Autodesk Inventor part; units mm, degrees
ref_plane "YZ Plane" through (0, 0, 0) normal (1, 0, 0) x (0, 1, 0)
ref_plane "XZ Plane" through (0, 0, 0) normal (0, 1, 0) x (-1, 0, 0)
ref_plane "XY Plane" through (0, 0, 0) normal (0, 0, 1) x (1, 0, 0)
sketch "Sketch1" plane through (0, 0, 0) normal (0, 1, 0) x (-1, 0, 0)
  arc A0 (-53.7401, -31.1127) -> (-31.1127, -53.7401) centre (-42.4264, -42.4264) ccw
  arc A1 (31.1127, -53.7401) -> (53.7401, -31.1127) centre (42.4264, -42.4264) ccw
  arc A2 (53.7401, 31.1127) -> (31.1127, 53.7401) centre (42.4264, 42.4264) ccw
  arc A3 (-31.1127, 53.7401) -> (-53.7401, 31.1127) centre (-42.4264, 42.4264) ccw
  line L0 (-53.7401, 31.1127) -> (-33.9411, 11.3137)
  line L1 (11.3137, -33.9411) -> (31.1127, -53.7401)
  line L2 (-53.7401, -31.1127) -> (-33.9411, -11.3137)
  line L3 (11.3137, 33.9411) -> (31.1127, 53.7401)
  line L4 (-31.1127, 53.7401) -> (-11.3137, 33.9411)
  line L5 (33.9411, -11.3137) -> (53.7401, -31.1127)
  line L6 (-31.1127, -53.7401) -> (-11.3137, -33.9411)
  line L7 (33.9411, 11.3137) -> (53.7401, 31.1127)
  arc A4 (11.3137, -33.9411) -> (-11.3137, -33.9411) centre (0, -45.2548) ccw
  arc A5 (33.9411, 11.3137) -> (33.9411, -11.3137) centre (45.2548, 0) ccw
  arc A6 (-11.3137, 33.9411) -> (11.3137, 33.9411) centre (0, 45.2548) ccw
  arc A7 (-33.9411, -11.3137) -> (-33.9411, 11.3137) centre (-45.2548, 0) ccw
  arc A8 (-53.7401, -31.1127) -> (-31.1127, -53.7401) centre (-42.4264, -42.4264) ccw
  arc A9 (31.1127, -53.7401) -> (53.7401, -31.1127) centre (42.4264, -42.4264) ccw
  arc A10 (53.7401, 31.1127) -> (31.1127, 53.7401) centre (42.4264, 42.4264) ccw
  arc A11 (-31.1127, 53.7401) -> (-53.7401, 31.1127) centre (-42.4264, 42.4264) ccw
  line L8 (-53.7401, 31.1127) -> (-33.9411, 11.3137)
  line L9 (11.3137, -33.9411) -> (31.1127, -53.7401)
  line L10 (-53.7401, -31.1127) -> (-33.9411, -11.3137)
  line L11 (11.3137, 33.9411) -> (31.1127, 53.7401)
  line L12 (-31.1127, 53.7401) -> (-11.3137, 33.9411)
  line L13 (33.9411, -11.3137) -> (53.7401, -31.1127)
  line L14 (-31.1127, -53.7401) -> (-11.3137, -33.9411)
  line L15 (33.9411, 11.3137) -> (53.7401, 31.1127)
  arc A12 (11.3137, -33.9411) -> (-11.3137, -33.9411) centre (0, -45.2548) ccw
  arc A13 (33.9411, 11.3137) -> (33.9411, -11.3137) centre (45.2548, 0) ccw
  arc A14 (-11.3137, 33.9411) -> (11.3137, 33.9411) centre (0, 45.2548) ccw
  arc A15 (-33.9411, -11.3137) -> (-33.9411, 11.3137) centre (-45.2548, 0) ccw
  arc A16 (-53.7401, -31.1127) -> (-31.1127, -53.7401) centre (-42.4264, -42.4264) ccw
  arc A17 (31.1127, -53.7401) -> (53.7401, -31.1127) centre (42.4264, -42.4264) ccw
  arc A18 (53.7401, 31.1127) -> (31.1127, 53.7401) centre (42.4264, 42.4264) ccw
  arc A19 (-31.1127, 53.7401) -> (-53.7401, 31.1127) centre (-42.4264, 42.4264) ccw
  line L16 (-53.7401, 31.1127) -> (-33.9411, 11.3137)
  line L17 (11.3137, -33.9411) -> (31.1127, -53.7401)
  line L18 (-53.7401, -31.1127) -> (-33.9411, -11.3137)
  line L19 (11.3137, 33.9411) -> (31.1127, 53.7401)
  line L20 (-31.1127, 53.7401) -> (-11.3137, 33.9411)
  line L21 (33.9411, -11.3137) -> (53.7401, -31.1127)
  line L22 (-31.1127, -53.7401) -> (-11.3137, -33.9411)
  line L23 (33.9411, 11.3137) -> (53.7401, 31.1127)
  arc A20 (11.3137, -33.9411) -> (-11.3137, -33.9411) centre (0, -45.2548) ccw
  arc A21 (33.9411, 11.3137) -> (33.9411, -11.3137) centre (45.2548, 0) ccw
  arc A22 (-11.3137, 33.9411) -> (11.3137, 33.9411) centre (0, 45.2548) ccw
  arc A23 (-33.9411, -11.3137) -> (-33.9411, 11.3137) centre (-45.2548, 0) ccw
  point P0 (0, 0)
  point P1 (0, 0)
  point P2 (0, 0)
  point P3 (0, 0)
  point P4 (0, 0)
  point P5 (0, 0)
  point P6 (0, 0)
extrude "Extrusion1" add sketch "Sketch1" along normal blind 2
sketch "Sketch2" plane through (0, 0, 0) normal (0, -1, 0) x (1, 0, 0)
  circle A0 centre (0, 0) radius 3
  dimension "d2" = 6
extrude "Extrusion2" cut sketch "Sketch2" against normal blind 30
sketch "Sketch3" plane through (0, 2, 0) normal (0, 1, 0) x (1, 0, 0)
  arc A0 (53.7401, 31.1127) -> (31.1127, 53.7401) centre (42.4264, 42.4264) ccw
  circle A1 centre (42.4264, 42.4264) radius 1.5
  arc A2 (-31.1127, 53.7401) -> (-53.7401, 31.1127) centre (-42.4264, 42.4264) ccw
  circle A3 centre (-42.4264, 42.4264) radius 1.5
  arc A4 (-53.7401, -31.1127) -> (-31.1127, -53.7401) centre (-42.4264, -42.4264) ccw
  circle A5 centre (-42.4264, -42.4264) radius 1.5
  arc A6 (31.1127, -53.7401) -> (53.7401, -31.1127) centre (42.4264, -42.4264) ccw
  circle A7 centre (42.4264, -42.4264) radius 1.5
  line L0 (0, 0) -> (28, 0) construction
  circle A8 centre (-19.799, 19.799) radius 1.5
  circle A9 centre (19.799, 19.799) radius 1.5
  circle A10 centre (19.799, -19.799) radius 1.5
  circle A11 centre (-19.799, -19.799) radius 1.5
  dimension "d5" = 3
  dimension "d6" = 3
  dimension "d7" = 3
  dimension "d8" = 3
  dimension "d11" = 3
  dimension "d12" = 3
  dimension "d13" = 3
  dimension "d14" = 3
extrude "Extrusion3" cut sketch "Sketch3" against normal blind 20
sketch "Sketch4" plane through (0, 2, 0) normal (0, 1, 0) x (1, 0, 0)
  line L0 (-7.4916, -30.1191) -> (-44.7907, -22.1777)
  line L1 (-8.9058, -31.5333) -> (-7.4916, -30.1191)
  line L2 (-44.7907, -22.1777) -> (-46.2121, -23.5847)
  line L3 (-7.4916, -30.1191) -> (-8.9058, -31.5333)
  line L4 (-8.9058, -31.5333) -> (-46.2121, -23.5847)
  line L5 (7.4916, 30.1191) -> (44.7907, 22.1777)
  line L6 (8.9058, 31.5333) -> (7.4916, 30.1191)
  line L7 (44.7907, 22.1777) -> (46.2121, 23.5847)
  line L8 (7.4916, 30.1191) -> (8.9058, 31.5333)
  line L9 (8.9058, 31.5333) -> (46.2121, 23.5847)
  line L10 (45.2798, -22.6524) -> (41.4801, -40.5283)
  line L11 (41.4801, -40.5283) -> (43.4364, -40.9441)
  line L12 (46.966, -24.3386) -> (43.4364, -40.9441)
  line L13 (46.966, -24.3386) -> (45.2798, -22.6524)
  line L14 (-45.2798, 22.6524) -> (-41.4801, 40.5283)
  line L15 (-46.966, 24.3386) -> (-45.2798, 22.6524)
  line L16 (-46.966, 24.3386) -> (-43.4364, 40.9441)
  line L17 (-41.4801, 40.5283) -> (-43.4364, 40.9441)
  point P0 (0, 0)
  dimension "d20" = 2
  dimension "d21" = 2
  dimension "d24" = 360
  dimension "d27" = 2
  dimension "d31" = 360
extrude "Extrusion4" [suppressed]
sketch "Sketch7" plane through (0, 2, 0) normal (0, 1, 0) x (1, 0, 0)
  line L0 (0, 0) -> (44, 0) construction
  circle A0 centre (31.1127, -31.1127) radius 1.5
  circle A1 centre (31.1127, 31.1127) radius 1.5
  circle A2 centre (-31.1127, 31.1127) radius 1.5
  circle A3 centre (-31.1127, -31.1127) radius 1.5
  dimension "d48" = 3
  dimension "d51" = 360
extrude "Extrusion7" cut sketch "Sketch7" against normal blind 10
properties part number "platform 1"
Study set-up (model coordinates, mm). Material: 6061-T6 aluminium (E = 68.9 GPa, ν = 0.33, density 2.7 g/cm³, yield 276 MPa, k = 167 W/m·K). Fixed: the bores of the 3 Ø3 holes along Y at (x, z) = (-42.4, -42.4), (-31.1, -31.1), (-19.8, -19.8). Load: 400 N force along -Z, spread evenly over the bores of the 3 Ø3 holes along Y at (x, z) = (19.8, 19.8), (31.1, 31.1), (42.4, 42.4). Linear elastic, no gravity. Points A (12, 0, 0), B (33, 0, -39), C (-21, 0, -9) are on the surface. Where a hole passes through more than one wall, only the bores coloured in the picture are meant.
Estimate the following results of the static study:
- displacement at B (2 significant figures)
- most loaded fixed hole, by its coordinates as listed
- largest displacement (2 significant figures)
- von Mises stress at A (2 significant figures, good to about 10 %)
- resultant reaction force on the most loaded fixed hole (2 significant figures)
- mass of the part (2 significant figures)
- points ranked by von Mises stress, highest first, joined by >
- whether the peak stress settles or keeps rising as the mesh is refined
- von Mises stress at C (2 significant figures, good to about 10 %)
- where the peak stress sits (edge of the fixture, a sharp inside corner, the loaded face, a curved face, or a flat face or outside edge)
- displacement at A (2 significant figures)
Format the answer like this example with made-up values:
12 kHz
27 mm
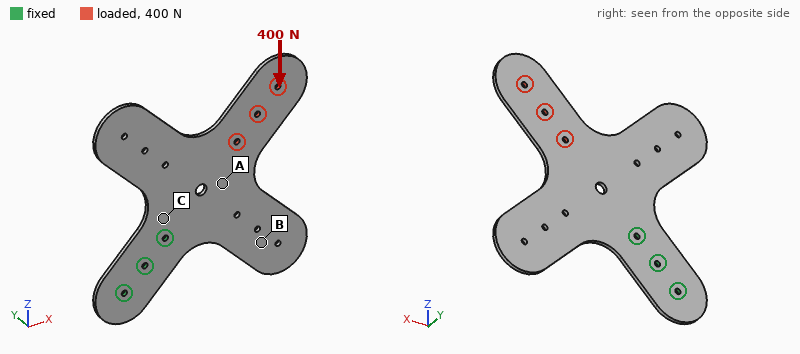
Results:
0.097 mm
(-19.8, -19.8)
0.19 mm
11 MPa
1.0 kN
45 g
C > A > B
keeps rising
22 MPa
edge of the fixture
0.064 mm
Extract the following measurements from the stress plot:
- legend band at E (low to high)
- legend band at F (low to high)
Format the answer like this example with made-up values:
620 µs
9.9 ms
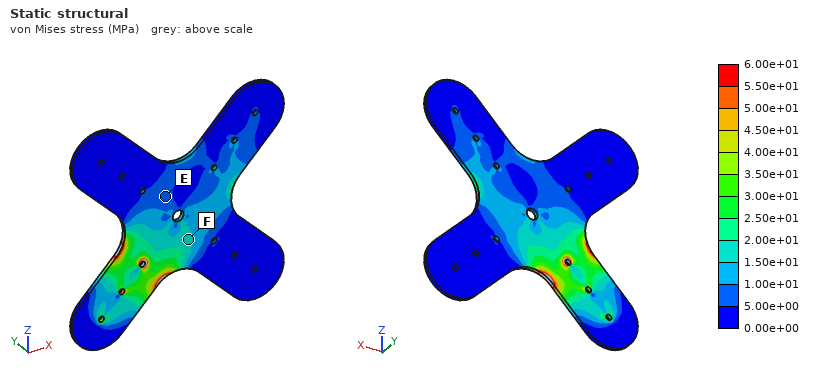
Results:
5.00e+00 to 1.00e+01 MPa
1.50e+01 to 2.00e+01 MPa
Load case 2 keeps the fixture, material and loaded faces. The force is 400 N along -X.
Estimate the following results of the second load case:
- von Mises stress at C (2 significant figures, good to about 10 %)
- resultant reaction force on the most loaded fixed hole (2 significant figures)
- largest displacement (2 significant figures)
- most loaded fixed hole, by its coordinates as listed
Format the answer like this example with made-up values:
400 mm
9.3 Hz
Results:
24 MPa
1.0 kN
0.19 mm
(-19.8, -19.8)
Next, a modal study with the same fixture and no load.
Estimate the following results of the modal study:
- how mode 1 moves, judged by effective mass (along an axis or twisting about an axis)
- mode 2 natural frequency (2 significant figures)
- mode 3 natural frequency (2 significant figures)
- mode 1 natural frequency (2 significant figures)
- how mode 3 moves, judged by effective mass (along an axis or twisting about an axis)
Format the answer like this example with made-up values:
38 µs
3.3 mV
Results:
along Y
230 Hz
370 Hz
180 Hz
along Y
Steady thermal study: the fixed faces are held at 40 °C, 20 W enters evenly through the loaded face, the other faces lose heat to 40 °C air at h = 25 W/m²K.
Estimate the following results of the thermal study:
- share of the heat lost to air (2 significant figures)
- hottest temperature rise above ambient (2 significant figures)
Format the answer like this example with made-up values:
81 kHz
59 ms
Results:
56 %
74 K
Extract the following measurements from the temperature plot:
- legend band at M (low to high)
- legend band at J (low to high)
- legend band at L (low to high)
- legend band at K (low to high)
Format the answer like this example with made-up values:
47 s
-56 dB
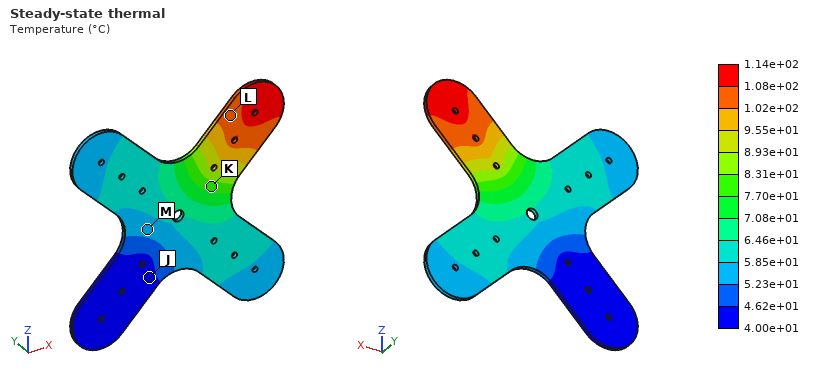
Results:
5.23e+01 to 5.85e+01 °C
4.00e+01 to 4.62e+01 °C
1.02e+02 to 1.08e+02 °C
7.70e+01 to 8.31e+01 °C
